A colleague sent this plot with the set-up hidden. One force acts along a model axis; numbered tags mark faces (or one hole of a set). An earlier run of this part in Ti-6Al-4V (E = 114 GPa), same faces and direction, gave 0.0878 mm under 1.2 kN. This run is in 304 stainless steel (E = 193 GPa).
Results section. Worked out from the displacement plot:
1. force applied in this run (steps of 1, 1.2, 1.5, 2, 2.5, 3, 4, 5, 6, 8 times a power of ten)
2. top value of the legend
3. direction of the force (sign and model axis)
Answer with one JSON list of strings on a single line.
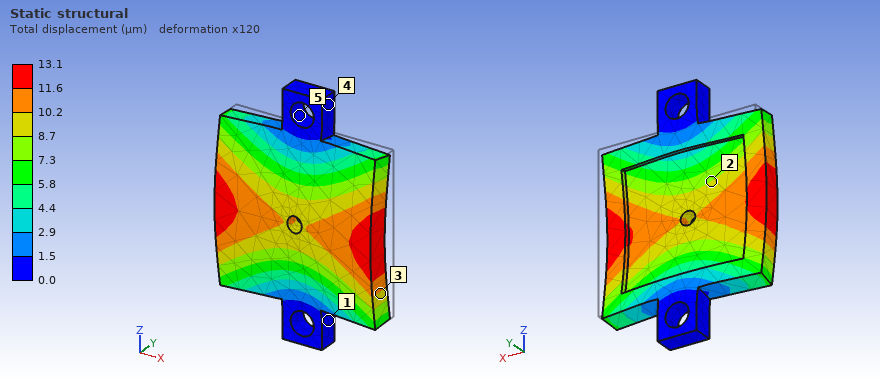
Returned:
["300 N", "13.1 µm", "-Y"]
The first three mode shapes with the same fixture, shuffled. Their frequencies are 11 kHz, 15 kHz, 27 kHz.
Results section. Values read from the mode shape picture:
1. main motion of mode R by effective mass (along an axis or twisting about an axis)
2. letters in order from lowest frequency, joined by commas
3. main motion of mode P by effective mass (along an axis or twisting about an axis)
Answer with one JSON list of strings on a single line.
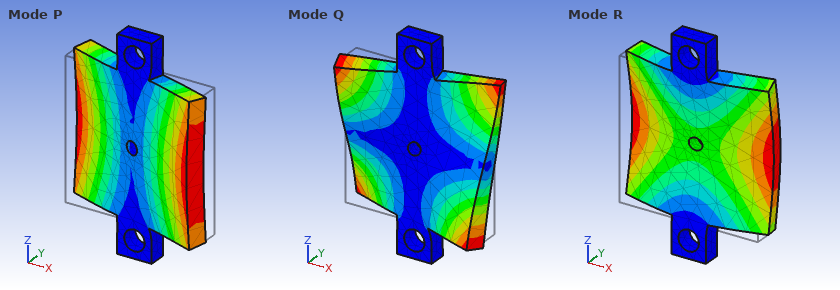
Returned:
["along Y", "P, R, Q", "twisting about Z"]
